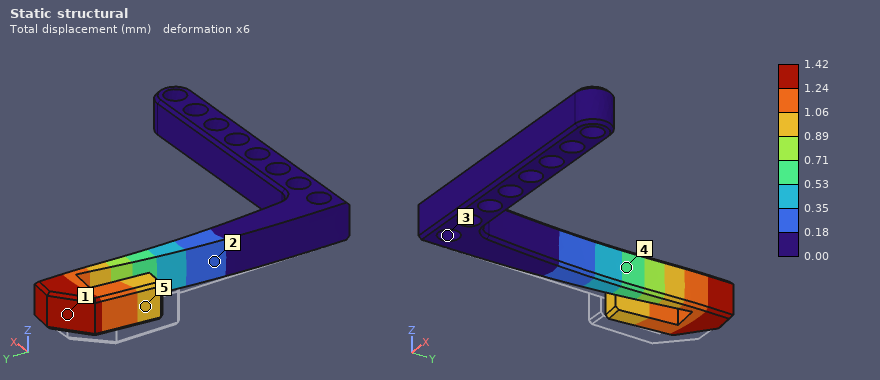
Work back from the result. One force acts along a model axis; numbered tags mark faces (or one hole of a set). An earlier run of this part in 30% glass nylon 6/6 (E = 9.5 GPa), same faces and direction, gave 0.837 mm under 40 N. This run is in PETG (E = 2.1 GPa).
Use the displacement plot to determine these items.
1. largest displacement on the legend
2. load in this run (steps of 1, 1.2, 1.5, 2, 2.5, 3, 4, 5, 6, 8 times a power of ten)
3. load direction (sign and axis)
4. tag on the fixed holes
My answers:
1.42 mm
15 N
+X
3
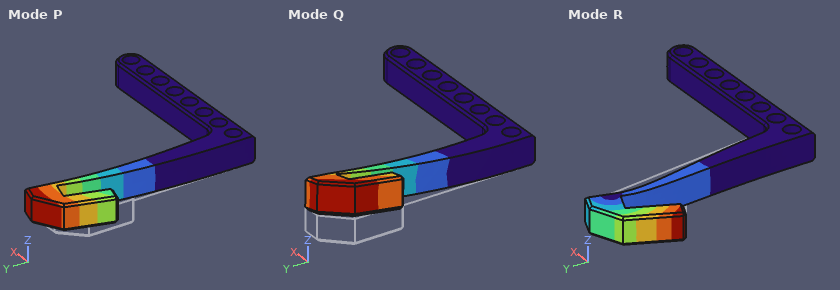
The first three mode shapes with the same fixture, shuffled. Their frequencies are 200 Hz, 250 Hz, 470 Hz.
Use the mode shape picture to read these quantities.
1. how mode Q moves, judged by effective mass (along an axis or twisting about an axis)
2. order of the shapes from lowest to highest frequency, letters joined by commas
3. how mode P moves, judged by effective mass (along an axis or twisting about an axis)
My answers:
along Z
P, Q, R
along X
